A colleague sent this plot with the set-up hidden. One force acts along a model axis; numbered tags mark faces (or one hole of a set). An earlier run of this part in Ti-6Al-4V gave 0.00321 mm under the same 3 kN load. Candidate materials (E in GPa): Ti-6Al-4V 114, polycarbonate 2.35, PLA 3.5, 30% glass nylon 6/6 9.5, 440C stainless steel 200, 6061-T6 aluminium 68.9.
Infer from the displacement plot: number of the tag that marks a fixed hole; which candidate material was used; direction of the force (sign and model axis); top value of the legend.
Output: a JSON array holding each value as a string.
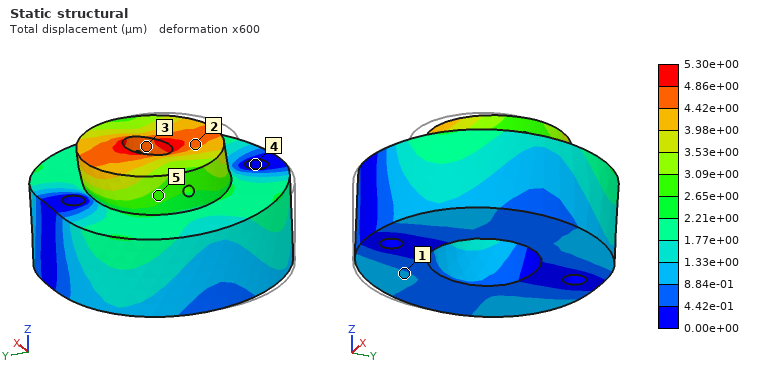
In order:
["4", "6061-T6 aluminium", "+Y", "5.30e+00 µm"]
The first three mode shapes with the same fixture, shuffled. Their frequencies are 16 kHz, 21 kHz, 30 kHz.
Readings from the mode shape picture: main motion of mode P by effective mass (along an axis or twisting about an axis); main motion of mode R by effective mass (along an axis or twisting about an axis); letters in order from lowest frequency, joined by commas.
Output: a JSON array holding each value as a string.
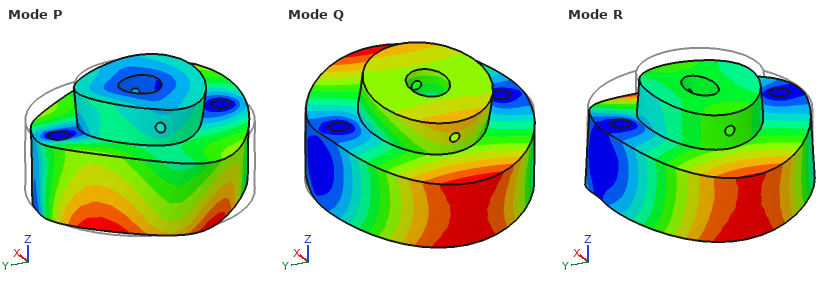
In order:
["twisting about Z", "along Z", "Q, R, P"]
